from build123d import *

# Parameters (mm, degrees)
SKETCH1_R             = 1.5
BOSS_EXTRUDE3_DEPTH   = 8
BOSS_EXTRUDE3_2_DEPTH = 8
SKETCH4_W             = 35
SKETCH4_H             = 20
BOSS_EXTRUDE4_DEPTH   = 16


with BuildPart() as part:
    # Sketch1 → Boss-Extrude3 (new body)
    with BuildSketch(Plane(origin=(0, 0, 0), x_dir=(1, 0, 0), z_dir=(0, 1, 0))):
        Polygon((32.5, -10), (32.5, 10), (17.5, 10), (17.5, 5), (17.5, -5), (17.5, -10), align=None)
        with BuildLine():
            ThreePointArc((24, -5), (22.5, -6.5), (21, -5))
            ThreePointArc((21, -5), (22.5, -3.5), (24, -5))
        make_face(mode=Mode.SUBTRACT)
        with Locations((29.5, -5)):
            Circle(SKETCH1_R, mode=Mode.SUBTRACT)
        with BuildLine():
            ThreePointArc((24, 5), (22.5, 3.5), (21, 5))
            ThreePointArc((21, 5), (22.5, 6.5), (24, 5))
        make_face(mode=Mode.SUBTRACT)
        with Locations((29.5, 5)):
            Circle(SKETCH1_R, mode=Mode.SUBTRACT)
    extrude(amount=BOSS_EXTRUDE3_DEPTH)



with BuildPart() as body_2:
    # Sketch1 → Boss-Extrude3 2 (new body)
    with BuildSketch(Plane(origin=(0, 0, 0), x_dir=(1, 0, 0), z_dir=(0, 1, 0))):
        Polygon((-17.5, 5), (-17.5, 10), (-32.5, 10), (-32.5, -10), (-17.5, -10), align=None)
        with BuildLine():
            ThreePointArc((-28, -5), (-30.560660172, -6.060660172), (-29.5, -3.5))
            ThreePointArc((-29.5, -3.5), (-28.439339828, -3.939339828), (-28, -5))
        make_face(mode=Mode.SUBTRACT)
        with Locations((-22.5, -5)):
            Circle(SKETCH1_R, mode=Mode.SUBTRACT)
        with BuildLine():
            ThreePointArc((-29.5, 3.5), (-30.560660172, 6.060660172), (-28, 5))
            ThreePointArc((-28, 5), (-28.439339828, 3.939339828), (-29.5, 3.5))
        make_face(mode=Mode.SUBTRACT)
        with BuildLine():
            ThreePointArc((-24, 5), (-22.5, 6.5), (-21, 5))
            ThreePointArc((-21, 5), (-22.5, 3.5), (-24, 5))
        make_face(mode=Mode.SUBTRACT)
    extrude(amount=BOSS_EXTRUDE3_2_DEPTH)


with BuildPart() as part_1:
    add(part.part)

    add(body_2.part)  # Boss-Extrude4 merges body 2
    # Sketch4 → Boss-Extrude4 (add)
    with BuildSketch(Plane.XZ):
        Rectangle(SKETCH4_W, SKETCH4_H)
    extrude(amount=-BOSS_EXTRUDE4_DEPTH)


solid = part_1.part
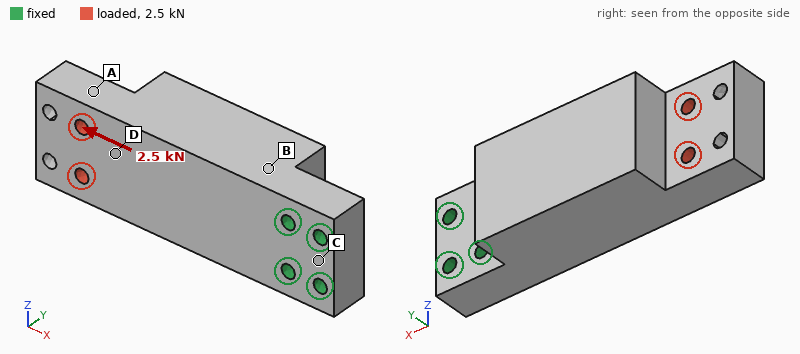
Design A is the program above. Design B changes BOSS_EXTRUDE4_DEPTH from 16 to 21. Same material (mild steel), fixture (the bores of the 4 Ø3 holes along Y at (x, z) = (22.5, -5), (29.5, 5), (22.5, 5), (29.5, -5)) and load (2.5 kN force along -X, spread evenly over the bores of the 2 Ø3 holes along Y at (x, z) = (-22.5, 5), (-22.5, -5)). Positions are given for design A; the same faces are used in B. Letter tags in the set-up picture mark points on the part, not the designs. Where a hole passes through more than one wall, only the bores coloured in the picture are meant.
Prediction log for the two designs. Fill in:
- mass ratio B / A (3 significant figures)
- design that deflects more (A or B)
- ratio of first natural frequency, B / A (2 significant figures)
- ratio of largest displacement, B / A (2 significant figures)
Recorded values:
1.23
A
0.91
0.88
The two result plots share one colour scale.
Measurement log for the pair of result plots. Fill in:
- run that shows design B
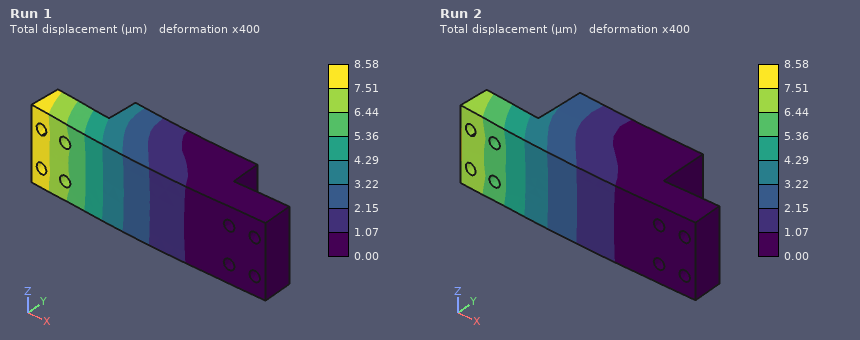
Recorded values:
Run 2
